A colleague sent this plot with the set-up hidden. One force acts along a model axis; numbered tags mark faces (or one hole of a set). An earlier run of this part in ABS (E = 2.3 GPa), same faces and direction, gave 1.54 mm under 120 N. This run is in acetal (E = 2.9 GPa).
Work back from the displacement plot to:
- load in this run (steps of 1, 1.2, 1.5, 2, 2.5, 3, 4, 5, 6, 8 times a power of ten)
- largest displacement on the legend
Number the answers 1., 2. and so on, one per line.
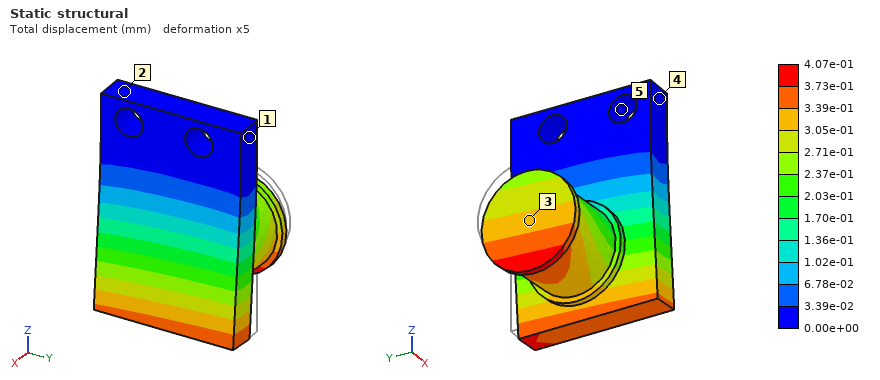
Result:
1. 40 N
2. 4.07e-01 mm
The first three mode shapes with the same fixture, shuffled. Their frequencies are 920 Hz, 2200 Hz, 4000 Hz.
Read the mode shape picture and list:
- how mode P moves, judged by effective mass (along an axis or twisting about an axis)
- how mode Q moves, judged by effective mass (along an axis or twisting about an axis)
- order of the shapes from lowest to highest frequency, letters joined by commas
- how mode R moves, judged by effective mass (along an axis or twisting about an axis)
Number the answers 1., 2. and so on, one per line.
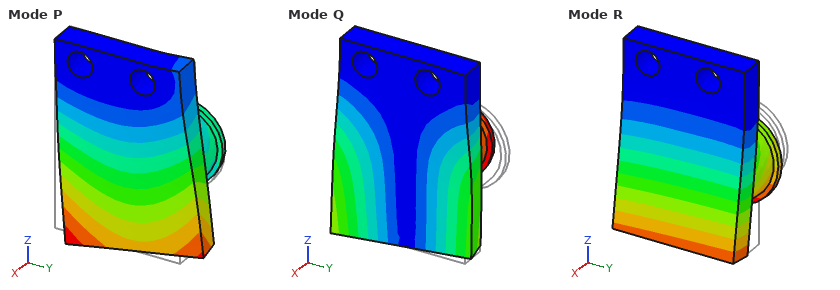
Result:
1. along Y
2. along Y
3. R, Q, P
4. along X
